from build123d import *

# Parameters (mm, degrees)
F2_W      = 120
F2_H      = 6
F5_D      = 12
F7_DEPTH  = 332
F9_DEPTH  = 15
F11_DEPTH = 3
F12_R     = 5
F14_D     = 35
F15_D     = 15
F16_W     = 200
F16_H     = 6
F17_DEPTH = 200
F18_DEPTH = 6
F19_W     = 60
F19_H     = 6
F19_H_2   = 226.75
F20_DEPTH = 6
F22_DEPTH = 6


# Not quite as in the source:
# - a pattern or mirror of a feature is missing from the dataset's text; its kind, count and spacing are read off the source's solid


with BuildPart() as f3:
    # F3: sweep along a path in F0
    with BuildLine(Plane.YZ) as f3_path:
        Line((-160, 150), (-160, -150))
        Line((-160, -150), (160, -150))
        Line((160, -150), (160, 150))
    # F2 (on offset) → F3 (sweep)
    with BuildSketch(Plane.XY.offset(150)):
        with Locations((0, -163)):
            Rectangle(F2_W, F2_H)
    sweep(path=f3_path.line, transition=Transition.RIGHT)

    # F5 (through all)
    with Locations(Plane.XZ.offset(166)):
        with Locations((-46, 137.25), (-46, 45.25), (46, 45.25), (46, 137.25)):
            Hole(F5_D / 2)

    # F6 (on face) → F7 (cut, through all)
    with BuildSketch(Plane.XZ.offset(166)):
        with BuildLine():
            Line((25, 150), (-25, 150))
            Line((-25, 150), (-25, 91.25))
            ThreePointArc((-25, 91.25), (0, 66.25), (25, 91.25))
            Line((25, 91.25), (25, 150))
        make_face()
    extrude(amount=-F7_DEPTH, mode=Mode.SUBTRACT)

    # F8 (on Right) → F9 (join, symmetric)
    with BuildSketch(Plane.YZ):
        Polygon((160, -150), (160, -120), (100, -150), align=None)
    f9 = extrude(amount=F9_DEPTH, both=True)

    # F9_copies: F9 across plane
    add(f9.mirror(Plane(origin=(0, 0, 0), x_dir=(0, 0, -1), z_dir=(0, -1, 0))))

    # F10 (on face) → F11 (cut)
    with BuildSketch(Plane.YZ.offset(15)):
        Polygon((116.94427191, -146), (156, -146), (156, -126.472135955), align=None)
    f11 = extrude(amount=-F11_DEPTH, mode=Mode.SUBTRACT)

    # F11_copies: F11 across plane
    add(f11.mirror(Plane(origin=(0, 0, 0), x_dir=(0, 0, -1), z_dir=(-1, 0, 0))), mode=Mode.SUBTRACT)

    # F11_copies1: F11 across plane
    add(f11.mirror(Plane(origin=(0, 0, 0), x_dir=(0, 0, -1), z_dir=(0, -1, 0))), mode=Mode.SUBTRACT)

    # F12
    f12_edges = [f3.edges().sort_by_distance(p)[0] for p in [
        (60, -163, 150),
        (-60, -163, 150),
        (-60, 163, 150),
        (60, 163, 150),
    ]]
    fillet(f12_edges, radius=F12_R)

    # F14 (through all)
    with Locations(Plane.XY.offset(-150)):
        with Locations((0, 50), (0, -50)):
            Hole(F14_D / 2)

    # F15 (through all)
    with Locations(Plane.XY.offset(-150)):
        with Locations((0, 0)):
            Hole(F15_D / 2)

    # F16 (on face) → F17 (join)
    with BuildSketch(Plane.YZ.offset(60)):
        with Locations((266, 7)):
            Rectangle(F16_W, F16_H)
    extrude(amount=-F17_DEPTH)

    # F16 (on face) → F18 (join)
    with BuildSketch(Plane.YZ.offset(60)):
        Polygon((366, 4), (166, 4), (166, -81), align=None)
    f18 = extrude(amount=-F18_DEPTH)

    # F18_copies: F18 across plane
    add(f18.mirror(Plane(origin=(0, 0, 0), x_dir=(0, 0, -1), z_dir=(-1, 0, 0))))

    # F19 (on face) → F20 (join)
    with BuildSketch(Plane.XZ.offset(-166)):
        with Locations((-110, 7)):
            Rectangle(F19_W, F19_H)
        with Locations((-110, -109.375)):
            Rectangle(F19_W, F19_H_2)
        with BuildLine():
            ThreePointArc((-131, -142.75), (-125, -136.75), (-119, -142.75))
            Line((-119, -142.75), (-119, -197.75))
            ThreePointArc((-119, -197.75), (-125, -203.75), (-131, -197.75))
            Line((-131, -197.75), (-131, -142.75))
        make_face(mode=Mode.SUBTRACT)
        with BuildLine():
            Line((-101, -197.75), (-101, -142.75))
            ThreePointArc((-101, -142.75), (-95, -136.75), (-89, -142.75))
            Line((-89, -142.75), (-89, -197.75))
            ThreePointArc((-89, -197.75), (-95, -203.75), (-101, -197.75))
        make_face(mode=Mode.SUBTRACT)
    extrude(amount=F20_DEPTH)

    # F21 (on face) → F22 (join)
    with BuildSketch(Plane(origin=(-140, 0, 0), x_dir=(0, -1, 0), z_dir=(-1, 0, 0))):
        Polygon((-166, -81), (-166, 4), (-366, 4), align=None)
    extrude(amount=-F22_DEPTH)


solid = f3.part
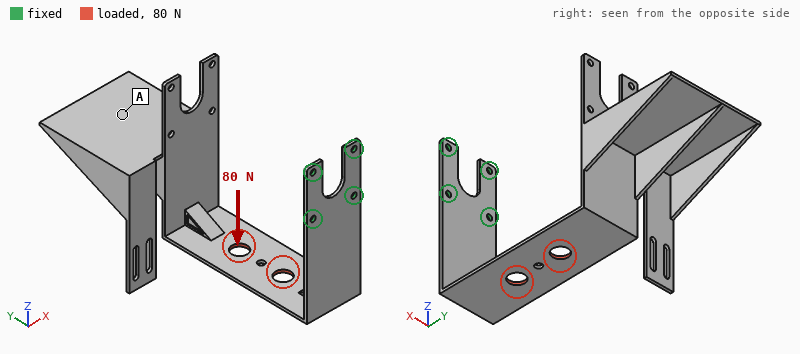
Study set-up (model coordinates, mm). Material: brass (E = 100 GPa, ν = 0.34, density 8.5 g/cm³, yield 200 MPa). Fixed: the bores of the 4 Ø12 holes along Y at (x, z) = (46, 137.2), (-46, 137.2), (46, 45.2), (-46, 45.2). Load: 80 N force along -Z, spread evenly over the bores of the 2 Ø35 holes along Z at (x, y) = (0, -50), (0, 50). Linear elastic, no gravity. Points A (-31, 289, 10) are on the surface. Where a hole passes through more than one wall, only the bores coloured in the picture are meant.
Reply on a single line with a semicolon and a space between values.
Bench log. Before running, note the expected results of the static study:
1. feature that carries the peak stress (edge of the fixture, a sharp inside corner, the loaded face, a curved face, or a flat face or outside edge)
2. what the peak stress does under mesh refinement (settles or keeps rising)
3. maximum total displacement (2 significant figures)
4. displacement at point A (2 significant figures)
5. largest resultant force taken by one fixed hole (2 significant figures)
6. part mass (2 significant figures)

edge of the fixture; keeps rising; 6.7 mm; 5.7 mm; 39 N; 9.6 kg
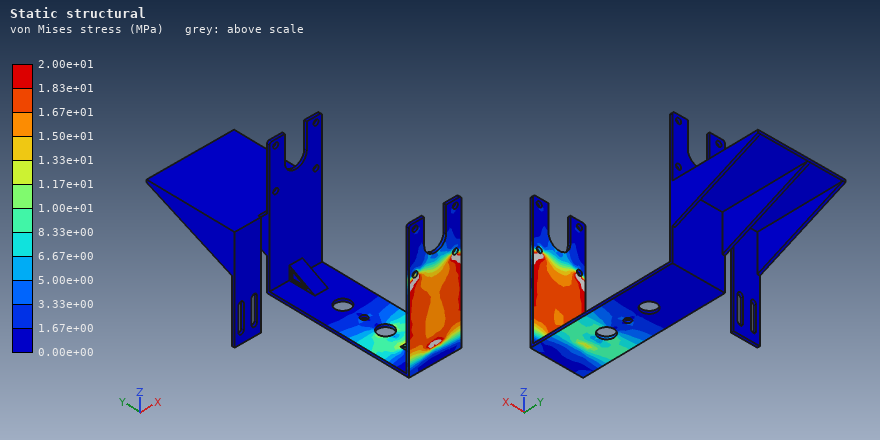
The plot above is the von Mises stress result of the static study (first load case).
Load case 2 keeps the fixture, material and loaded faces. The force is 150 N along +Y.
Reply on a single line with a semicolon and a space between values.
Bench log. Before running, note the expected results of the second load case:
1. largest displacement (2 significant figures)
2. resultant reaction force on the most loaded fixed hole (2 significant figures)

6.9 mm; 100 N
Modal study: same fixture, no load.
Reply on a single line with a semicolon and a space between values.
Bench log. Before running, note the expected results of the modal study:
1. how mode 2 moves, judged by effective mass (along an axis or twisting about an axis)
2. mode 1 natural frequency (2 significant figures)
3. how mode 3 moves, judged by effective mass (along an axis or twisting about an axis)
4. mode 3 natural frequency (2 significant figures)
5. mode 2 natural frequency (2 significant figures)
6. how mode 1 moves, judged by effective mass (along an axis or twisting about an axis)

along X; 4.6 Hz; along Y; 15 Hz; 7.3 Hz; along Z
